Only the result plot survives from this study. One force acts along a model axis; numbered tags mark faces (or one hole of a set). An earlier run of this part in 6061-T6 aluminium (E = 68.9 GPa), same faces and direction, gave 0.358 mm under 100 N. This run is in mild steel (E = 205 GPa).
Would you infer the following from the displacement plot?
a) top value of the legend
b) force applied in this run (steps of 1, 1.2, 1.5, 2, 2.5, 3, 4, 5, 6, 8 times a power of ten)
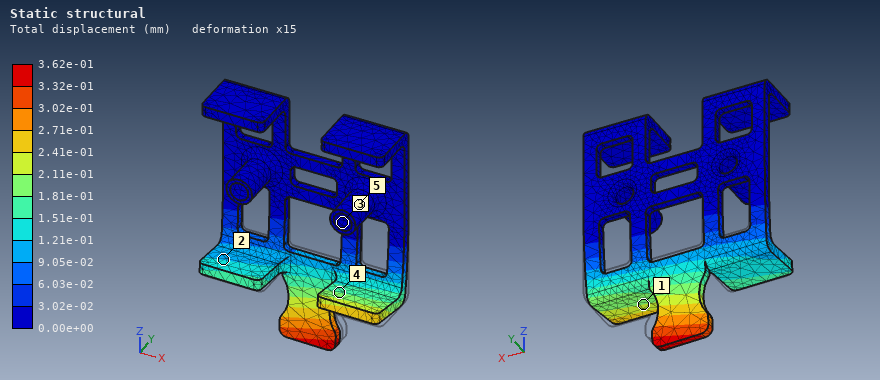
3.62e-01 mm
300 N
